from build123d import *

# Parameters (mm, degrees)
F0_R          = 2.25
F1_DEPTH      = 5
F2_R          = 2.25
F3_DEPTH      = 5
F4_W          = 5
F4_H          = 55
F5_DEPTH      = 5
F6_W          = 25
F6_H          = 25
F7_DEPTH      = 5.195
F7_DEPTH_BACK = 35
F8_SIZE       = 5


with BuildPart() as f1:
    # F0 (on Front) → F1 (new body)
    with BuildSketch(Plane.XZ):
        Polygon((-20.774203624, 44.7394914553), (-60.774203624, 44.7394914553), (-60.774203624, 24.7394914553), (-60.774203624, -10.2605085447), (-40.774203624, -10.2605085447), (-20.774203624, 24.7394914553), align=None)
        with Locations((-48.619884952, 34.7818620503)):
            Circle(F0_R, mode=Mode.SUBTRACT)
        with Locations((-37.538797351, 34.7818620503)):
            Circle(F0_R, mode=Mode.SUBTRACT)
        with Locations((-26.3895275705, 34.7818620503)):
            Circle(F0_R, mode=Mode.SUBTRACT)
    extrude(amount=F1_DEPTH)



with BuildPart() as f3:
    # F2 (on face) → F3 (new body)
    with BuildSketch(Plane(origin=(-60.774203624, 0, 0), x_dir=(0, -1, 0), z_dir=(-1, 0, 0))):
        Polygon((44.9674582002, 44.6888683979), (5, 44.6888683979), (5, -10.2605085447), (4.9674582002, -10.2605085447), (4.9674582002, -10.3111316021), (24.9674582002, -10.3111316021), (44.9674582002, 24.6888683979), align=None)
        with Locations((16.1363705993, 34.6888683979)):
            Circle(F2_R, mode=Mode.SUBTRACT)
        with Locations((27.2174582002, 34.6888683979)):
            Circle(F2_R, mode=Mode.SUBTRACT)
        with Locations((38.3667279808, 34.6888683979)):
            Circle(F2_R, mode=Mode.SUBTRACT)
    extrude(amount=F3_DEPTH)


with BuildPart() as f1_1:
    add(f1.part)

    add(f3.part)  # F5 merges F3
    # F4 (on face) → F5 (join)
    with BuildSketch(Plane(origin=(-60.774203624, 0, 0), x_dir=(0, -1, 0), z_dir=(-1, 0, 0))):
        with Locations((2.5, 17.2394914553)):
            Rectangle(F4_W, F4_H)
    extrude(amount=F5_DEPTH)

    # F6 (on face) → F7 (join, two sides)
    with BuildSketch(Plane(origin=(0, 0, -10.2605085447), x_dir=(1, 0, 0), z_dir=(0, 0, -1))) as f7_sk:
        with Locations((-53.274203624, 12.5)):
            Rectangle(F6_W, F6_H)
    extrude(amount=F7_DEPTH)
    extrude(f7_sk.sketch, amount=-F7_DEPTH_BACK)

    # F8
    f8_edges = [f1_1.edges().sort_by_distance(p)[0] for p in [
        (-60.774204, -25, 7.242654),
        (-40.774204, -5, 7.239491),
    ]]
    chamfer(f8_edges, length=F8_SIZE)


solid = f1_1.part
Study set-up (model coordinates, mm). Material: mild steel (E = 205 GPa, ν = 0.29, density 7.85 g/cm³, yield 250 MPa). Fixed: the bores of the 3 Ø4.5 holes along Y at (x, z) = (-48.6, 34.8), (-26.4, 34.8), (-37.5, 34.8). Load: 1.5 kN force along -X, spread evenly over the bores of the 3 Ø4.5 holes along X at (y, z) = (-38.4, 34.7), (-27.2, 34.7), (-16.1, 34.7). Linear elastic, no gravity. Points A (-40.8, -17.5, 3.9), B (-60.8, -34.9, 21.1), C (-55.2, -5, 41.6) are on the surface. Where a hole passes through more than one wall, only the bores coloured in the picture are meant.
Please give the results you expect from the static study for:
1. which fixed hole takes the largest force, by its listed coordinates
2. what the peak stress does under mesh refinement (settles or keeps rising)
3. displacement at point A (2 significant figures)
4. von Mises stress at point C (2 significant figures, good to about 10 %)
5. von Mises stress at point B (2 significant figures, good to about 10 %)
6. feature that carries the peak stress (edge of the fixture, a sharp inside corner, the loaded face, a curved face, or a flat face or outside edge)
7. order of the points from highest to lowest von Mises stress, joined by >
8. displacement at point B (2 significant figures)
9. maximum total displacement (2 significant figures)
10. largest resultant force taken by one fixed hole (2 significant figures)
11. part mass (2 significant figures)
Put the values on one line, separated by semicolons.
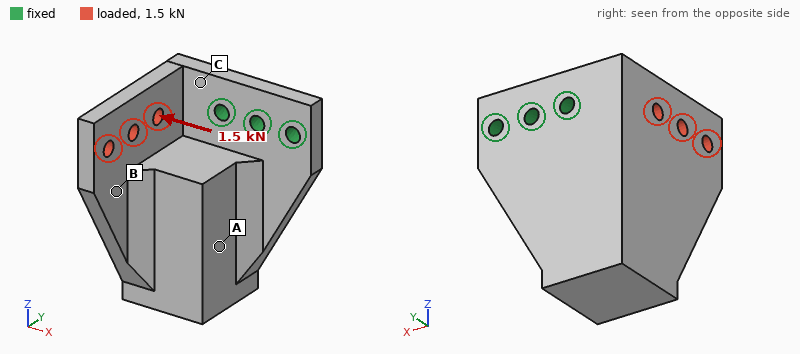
(-48.6, 34.8); keeps rising; 0.028 mm; 94 MPa; 58 MPa; edge of the fixture; C > B > A; 0.072 mm; 0.14 mm; 1.8 kN; 290 g
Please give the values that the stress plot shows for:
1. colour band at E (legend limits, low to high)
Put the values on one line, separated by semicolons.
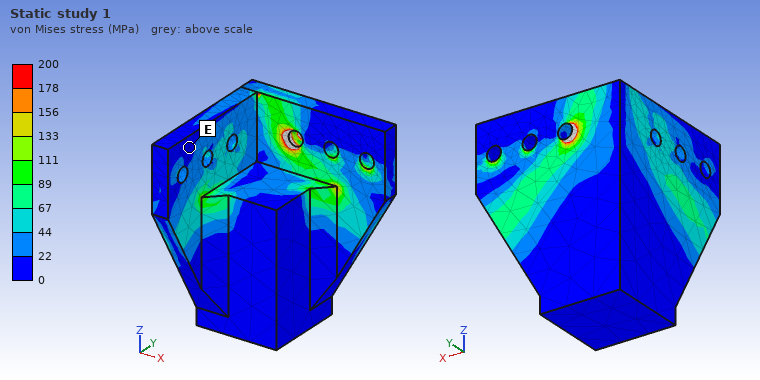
0 to 22 MPa
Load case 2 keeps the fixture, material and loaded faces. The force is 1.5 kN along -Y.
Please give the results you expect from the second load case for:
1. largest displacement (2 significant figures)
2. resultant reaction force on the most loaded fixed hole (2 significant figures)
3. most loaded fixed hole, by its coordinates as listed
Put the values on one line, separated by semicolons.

46 µm; 2.2 kN; (-48.6, 34.8)
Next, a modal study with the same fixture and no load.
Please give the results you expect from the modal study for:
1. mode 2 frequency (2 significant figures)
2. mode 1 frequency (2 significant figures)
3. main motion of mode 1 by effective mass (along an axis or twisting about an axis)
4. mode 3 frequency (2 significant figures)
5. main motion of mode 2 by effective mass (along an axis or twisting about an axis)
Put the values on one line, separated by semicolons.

2700 Hz; 990 Hz; along Y; 4800 Hz; along X
